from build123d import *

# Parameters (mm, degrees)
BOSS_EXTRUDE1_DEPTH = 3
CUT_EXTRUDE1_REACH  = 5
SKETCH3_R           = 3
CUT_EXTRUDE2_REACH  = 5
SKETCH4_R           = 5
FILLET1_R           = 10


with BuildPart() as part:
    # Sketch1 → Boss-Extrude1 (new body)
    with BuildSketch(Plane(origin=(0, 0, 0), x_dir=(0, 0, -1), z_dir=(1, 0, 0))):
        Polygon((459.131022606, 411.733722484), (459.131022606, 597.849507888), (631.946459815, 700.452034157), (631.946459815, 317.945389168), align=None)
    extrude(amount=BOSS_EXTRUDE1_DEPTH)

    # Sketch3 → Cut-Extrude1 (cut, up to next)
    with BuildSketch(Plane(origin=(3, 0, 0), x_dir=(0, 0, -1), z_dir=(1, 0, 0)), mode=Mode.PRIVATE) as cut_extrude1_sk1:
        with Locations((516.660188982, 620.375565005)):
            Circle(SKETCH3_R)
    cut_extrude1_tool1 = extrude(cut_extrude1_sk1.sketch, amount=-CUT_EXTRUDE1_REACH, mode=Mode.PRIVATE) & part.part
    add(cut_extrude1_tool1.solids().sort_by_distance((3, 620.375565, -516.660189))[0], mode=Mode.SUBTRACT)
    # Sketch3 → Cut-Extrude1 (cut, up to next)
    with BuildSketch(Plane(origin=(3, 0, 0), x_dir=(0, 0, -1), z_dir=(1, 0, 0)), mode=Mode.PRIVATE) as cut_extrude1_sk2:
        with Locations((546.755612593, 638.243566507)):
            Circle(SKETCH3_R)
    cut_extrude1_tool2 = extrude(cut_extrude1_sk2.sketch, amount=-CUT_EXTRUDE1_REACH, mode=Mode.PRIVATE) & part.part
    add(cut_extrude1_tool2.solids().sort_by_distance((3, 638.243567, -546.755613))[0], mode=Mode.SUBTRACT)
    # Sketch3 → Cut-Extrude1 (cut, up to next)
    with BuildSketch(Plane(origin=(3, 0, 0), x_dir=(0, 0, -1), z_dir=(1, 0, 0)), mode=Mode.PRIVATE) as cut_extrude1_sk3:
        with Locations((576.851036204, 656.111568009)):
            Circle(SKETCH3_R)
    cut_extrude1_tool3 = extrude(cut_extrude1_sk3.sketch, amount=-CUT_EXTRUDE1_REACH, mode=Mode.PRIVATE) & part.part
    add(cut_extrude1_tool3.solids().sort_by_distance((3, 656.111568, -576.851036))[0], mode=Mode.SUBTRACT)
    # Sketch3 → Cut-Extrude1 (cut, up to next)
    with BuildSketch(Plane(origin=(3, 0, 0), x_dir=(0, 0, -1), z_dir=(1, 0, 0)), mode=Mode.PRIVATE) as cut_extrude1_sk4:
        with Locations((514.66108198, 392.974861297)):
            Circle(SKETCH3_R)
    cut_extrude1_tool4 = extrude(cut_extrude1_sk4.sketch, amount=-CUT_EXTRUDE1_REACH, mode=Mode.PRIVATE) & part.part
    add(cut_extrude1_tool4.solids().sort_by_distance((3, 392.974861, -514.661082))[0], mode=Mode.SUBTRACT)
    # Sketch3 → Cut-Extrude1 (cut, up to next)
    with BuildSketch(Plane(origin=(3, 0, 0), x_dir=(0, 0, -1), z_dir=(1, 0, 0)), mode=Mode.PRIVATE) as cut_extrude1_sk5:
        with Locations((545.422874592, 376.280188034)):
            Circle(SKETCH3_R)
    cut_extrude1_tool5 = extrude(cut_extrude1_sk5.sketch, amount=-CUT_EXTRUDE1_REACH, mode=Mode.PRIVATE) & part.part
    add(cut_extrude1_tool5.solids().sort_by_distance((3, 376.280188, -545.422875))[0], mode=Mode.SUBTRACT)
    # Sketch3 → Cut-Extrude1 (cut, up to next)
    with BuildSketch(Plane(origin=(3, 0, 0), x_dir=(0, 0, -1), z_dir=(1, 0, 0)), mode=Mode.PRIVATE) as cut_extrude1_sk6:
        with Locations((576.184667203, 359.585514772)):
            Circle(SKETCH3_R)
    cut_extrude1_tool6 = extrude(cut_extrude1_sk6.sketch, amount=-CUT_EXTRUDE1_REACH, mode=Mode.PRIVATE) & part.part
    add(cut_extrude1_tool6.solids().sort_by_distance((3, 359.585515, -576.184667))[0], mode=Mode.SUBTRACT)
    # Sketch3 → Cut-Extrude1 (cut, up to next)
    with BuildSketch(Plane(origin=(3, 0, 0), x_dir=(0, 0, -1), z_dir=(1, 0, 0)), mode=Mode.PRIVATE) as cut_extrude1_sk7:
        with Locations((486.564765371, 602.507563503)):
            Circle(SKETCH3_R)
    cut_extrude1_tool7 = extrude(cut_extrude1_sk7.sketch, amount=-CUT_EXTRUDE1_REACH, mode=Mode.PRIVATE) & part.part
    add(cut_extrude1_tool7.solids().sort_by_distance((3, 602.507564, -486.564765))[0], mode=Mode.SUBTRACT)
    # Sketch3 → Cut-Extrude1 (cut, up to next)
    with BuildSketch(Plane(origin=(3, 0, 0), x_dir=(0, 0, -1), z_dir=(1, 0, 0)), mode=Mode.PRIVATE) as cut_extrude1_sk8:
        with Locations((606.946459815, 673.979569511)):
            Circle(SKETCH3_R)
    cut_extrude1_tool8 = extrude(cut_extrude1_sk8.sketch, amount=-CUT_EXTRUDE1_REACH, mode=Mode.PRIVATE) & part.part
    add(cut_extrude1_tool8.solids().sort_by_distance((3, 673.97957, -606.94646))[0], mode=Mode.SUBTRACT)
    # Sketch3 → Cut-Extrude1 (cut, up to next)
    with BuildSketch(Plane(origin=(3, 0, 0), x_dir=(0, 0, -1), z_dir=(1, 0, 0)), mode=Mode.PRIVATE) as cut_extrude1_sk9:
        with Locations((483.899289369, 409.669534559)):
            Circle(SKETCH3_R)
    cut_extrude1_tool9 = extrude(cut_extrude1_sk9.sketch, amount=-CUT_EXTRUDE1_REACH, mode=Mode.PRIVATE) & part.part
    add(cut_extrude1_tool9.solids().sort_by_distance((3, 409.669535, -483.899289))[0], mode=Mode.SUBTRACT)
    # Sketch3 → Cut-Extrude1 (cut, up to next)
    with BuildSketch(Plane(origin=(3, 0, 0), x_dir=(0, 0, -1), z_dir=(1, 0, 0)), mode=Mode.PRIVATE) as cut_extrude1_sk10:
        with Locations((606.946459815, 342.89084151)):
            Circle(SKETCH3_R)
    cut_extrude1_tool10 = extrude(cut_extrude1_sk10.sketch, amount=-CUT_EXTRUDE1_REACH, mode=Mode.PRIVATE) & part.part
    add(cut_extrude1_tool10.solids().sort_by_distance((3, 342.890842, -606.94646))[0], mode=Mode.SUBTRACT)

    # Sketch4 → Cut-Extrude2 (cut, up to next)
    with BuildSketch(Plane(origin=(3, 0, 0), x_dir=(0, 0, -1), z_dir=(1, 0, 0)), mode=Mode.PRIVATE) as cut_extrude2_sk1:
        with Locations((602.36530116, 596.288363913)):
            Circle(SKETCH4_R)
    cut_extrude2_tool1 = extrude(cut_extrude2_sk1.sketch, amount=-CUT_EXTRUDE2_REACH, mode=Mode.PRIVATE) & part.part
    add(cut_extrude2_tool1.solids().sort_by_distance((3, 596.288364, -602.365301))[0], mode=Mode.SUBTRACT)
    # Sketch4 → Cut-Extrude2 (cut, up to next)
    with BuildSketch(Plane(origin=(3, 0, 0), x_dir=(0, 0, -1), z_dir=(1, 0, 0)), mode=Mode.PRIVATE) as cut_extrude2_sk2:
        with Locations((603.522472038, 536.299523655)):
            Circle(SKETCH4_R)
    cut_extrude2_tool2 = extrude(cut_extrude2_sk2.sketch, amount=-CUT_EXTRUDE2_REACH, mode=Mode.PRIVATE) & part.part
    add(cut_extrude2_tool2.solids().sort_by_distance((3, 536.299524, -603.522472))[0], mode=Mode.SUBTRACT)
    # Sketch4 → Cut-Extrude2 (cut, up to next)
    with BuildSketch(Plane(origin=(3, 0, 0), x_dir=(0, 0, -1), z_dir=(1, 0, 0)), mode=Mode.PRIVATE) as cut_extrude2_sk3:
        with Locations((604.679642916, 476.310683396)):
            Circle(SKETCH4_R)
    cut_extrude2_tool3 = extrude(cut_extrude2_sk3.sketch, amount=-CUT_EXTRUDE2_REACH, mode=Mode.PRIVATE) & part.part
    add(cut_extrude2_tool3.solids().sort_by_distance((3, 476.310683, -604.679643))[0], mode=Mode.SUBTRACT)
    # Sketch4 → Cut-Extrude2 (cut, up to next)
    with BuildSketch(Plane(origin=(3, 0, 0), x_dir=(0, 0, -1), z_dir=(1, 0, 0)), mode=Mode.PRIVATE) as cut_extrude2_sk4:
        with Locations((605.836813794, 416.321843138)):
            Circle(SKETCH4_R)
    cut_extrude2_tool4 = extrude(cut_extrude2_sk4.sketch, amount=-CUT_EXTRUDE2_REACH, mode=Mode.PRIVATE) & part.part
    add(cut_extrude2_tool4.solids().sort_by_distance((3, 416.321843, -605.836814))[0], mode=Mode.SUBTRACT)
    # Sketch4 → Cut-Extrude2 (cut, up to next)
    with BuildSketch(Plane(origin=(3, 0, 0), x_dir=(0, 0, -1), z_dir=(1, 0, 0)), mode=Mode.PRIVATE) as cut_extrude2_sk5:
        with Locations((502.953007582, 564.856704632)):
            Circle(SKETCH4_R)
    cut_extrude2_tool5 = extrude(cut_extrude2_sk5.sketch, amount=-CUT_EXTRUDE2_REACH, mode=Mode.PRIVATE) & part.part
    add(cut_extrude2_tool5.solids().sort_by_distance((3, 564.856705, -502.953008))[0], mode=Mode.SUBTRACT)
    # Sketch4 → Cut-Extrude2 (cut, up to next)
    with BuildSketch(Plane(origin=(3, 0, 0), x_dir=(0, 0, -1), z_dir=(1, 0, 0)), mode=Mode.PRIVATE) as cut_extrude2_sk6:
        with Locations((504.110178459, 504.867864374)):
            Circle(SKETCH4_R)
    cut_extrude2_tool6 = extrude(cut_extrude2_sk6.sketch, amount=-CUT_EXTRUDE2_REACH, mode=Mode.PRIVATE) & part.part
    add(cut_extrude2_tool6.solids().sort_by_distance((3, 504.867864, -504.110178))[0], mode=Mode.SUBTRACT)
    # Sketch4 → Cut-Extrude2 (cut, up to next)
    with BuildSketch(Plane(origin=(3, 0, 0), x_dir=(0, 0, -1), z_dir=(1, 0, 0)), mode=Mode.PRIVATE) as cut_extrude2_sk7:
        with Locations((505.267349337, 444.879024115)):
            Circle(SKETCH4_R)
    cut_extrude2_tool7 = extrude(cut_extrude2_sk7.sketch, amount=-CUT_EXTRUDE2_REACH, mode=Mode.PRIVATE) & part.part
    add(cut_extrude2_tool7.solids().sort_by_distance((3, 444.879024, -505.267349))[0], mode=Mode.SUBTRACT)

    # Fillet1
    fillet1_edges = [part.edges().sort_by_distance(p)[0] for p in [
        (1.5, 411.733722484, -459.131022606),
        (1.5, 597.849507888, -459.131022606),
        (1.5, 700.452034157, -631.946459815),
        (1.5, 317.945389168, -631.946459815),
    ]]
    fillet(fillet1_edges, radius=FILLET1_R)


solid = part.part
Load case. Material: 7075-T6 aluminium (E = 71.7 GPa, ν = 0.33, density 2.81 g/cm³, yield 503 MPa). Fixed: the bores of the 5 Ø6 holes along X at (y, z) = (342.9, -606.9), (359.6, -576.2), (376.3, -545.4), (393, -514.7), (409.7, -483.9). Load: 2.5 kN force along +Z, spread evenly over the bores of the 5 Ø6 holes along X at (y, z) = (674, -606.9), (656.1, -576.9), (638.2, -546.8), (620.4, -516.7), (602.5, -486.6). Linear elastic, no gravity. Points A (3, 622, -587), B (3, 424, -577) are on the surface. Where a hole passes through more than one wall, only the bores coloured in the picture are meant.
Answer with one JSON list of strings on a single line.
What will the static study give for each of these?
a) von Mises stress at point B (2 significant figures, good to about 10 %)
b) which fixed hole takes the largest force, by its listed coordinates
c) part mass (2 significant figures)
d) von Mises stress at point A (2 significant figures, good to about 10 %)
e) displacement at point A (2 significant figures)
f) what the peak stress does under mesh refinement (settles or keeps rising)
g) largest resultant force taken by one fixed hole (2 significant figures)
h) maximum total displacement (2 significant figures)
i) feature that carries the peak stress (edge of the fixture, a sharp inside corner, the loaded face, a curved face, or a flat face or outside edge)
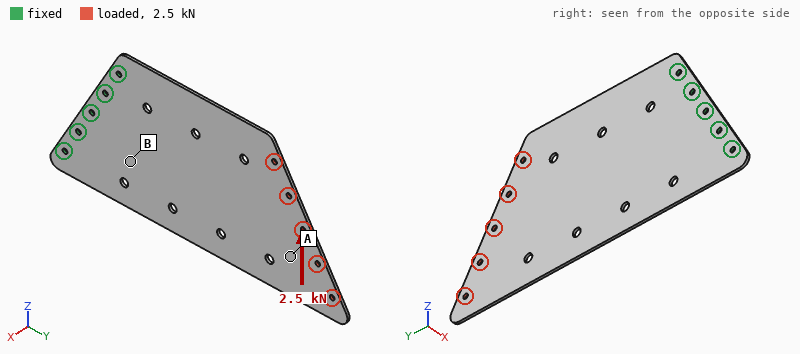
["19 MPa", "(409.7, -483.9)", "410 g", "6.8 MPa", "0.24 mm", "keeps rising", "5.0 kN", "0.35 mm", "edge of the fixture"]
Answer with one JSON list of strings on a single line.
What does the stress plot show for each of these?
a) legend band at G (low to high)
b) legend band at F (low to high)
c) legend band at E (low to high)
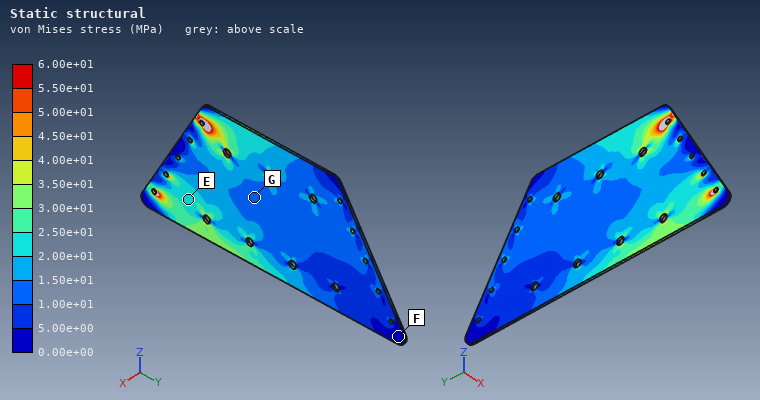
["1.00e+01 to 1.50e+01 MPa", "0.00e+00 to 5.00e+00 MPa", "2.00e+01 to 2.50e+01 MPa"]
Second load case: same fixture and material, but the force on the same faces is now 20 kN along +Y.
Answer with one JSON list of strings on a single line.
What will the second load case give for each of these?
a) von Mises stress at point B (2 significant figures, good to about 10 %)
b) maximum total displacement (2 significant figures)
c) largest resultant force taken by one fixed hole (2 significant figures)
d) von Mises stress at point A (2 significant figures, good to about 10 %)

["41 MPa", "0.22 mm", "4.4 kN", "42 MPa"]
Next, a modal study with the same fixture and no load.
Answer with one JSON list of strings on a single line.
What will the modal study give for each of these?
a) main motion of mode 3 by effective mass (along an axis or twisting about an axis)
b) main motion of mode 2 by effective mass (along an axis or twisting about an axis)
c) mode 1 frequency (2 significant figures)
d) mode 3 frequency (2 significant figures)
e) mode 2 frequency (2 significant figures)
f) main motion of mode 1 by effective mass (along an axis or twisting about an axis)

["along X", "twisting about Y", "35 Hz", "190 Hz", "130 Hz", "along X"]
